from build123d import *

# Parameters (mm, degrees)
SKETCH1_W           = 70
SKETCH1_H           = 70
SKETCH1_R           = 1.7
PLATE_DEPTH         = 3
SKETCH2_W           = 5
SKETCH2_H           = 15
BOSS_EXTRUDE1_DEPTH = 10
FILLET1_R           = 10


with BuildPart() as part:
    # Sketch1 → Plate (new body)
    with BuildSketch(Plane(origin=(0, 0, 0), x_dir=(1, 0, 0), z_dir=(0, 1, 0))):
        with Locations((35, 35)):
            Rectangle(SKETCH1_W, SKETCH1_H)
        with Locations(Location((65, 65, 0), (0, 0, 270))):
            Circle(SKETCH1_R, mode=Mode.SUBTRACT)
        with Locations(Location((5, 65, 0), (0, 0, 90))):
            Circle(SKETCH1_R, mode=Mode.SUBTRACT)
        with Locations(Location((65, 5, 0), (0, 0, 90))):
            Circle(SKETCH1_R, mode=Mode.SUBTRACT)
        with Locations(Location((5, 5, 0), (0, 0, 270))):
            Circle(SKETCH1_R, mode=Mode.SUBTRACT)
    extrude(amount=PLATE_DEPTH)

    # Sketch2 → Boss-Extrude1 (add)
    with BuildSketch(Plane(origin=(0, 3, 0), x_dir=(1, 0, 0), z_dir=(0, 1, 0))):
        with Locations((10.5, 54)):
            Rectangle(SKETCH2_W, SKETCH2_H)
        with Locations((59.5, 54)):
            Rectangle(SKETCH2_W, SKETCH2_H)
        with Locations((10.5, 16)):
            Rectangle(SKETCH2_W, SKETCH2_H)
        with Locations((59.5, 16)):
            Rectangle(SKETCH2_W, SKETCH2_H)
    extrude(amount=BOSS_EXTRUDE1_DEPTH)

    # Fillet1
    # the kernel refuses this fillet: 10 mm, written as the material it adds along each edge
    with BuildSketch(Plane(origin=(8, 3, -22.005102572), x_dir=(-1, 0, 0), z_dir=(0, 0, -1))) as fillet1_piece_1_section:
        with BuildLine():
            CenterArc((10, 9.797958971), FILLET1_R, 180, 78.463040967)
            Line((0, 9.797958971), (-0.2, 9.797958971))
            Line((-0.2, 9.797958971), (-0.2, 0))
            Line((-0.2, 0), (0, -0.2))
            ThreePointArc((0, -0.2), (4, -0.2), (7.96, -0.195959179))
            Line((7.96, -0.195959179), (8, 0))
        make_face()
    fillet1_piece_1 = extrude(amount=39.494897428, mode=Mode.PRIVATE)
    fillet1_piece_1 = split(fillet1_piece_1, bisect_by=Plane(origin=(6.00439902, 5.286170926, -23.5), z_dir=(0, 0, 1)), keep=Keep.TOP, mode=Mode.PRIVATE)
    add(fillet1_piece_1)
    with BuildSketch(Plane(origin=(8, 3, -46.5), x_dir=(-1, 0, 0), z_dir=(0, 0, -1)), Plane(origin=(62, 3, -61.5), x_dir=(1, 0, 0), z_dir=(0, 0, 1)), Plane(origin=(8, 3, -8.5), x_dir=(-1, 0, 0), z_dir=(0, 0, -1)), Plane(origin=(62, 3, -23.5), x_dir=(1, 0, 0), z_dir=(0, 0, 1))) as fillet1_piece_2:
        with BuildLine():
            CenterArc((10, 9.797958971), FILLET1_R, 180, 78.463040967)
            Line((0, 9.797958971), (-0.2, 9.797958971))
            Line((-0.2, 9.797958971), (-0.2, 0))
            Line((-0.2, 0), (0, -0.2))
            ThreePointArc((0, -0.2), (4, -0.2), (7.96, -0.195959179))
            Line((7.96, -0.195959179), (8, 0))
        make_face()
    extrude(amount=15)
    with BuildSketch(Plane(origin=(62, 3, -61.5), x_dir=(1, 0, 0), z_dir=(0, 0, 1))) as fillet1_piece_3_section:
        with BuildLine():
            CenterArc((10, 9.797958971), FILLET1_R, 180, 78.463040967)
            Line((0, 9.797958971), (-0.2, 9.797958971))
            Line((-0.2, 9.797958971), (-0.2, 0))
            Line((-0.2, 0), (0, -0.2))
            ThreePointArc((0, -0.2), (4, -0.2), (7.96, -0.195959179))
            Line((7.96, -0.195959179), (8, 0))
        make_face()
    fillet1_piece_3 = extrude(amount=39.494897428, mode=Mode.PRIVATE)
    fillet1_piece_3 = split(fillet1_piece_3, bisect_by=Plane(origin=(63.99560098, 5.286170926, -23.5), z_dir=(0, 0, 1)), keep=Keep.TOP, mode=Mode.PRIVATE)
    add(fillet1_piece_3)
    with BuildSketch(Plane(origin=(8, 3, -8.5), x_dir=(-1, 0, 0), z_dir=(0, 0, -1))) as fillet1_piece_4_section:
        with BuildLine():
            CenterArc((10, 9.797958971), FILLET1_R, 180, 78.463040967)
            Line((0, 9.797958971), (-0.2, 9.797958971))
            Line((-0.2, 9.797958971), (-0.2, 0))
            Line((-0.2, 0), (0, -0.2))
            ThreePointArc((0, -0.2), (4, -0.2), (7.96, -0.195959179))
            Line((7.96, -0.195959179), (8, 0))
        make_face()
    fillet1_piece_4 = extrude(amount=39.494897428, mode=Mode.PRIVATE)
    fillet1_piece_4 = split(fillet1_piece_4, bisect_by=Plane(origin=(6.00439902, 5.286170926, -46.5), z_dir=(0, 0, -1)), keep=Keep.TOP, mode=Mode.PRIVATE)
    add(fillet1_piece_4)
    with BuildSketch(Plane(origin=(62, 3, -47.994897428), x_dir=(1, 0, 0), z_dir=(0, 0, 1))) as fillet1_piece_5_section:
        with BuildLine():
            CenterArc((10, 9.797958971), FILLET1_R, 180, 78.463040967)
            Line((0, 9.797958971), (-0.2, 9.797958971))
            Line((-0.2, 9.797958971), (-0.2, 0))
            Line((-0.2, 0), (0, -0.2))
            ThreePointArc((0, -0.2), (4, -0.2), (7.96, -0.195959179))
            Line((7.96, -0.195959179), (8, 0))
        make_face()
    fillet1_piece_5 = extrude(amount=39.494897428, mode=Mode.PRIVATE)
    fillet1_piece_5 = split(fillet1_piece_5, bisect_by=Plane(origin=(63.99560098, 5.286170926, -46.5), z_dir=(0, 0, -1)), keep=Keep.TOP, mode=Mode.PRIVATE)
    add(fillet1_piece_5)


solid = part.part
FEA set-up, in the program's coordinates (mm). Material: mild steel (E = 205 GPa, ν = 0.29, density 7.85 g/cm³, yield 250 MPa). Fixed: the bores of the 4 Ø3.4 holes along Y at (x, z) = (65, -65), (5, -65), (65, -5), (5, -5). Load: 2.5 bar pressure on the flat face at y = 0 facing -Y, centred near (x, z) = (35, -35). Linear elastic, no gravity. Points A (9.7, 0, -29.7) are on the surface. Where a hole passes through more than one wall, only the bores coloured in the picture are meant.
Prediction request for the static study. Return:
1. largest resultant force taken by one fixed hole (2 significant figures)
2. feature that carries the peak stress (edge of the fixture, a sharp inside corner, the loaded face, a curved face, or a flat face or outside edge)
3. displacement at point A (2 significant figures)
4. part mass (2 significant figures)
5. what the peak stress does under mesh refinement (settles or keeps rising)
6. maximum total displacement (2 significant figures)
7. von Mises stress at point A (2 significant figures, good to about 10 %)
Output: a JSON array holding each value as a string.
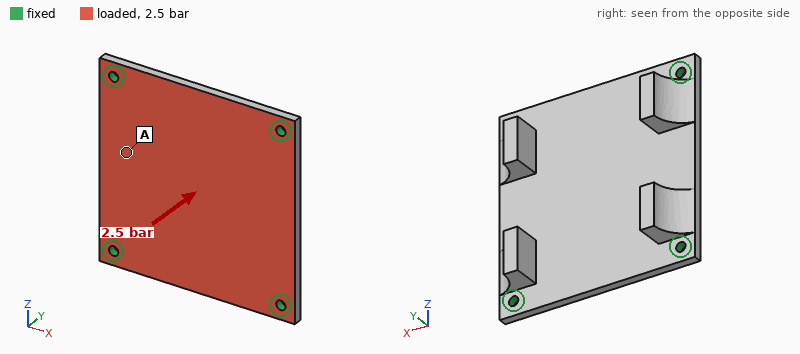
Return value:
["310 N", "edge of the fixture", "29 µm", "150 g", "keeps rising", "45 µm", "28 MPa"]
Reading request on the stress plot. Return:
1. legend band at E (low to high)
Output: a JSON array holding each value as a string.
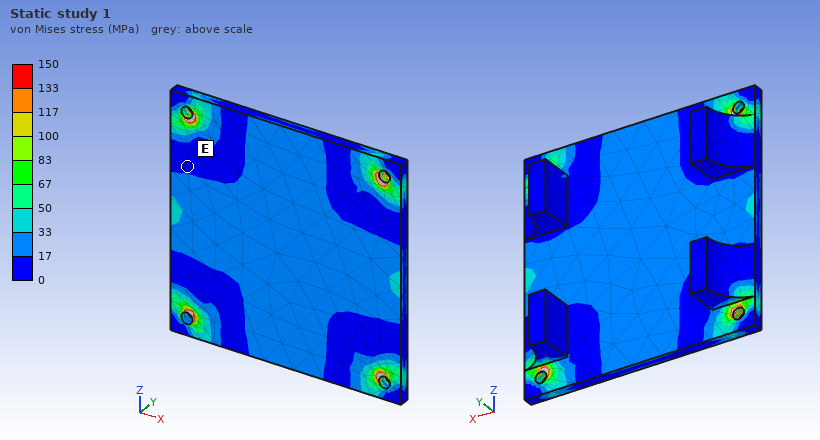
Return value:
["0 to 17 MPa"]
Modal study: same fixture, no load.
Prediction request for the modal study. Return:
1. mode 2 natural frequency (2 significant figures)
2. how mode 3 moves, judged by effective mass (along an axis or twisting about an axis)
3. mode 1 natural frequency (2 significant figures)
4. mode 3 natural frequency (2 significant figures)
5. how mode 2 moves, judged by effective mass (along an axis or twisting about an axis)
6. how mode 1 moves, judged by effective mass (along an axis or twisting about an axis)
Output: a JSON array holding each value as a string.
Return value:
["4600 Hz", "twisting about X", "2800 Hz", "5000 Hz", "twisting about Z", "along Y"]
